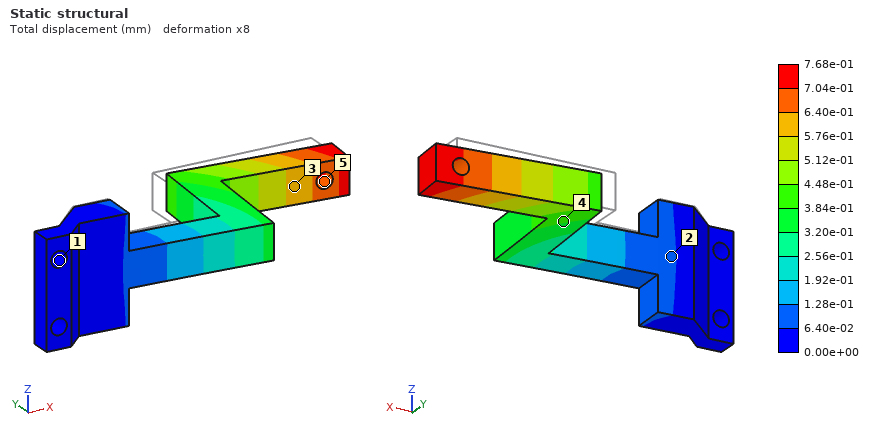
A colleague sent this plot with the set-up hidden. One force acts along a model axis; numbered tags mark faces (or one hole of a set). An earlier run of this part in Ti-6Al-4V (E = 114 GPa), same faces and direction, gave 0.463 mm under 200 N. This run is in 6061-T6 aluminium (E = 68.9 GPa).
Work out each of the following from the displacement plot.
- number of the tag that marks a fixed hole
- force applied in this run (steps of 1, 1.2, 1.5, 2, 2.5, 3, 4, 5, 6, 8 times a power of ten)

1
200 N
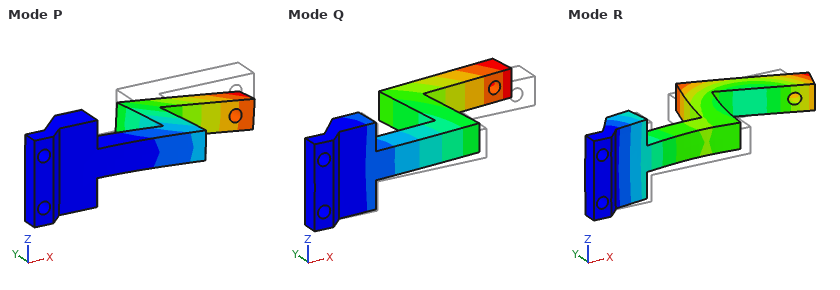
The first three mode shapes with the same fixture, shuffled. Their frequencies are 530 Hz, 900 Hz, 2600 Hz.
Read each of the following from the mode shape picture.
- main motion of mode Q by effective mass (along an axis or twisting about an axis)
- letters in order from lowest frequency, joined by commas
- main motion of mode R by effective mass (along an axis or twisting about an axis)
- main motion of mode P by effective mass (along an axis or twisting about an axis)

along Y
Q, P, R
along Y
along Z
